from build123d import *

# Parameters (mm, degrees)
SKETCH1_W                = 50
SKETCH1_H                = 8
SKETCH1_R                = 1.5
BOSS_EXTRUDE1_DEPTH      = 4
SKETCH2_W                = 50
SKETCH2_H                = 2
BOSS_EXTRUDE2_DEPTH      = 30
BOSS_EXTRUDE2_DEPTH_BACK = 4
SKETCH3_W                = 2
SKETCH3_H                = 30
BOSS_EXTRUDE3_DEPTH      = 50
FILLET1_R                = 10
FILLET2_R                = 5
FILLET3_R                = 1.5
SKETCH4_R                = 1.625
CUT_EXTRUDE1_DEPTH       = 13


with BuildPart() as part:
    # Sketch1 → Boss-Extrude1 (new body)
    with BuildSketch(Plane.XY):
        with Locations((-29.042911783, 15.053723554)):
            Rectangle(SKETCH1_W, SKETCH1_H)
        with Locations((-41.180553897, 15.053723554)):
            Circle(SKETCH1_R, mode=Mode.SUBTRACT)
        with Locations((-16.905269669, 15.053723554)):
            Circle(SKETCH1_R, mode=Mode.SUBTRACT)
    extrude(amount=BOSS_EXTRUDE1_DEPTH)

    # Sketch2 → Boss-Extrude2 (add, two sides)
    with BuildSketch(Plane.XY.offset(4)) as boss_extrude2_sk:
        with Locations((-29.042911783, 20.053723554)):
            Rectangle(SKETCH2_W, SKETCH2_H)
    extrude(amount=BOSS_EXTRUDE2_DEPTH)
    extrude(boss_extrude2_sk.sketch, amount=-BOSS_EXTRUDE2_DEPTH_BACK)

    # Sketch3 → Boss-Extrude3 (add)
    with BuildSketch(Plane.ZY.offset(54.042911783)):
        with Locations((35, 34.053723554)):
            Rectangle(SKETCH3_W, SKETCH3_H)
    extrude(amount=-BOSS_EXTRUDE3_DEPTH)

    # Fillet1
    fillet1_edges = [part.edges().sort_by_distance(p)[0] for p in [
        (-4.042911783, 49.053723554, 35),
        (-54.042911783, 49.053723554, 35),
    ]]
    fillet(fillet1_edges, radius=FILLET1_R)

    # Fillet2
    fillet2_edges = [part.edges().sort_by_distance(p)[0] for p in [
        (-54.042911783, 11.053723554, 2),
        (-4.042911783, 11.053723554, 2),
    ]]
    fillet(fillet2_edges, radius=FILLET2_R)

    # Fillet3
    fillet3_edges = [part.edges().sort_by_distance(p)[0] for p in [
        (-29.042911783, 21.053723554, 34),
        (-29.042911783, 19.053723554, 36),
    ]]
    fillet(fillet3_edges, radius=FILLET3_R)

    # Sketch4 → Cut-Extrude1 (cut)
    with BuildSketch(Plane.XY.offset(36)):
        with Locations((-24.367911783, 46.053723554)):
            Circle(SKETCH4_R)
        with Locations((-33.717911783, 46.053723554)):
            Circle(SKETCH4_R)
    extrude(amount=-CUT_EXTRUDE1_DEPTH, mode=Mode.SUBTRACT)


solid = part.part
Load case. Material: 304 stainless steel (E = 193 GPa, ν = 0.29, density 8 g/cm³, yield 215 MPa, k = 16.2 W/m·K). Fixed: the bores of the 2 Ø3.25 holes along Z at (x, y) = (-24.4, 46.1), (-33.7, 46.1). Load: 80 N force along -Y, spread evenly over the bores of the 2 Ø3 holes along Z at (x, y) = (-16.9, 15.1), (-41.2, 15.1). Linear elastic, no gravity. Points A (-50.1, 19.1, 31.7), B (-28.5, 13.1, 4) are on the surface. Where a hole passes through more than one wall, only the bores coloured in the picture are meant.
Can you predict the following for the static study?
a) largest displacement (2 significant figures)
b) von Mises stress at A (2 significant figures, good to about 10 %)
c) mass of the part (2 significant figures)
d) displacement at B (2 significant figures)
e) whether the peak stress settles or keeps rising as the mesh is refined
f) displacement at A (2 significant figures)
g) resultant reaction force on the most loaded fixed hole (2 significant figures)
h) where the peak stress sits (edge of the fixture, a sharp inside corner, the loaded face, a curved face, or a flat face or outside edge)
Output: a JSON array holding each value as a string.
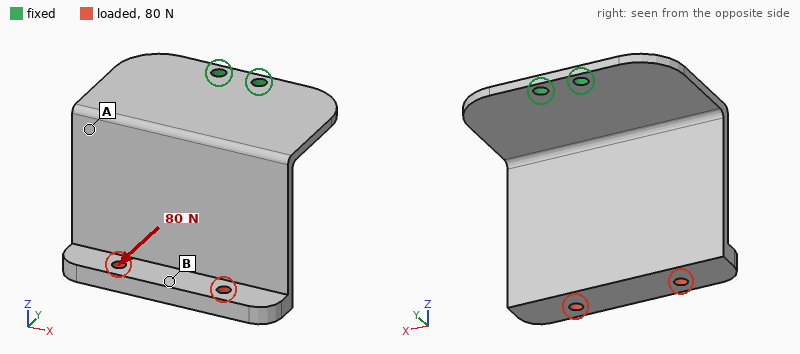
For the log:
["0.63 mm", "59 MPa", "62 g", "0.55 mm", "keeps rising", "0.18 mm", "40 N", "edge of the fixture"]
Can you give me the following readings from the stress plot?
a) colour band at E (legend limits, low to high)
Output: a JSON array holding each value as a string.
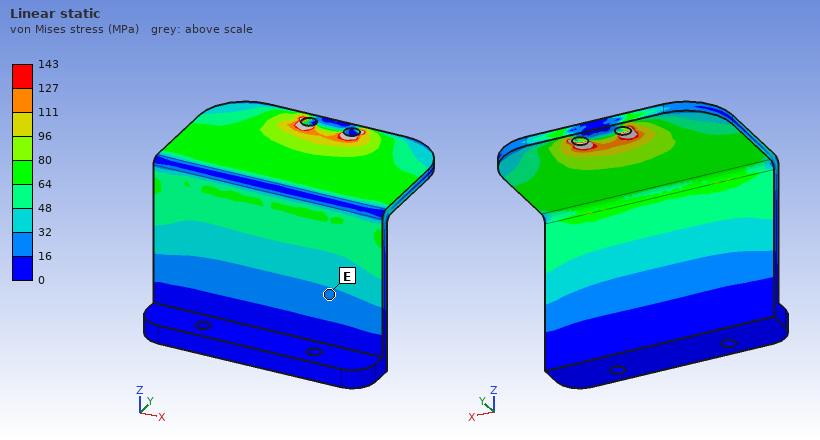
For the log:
["16 to 32 MPa"]
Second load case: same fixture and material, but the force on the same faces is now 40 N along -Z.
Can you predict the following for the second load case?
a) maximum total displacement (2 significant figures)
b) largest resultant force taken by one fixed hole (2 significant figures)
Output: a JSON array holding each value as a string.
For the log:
["0.17 mm", "20 N"]
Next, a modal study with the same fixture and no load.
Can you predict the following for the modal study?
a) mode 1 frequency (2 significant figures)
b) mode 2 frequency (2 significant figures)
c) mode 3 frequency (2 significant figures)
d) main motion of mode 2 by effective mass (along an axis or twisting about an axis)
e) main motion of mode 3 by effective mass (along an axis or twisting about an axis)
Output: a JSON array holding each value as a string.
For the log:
["370 Hz", "580 Hz", "1200 Hz", "along X", "along Z"]
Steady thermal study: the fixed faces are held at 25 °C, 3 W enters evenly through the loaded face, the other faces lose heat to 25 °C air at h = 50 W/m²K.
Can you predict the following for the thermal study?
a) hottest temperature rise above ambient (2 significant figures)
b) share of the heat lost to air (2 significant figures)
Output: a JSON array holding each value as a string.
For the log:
["28 K", "97 %"]
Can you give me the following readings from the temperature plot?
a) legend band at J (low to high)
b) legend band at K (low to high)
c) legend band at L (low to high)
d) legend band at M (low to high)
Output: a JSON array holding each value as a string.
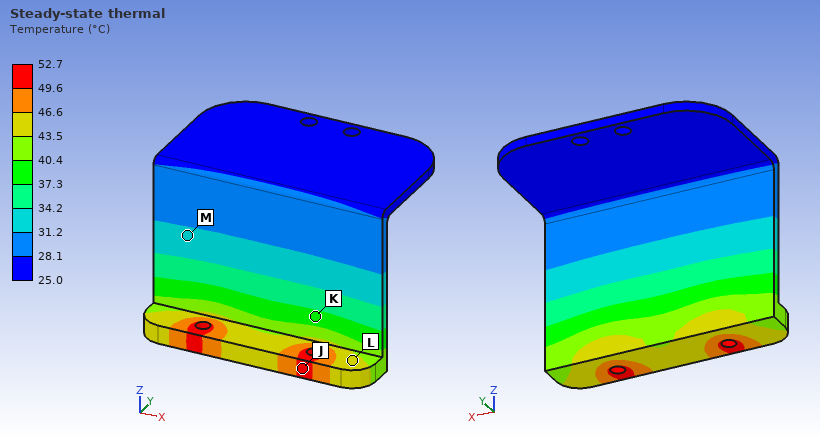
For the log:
["49.6 to 52.7 °C", "37.3 to 40.4 °C", "43.5 to 46.6 °C", "31.2 to 34.2 °C"]
